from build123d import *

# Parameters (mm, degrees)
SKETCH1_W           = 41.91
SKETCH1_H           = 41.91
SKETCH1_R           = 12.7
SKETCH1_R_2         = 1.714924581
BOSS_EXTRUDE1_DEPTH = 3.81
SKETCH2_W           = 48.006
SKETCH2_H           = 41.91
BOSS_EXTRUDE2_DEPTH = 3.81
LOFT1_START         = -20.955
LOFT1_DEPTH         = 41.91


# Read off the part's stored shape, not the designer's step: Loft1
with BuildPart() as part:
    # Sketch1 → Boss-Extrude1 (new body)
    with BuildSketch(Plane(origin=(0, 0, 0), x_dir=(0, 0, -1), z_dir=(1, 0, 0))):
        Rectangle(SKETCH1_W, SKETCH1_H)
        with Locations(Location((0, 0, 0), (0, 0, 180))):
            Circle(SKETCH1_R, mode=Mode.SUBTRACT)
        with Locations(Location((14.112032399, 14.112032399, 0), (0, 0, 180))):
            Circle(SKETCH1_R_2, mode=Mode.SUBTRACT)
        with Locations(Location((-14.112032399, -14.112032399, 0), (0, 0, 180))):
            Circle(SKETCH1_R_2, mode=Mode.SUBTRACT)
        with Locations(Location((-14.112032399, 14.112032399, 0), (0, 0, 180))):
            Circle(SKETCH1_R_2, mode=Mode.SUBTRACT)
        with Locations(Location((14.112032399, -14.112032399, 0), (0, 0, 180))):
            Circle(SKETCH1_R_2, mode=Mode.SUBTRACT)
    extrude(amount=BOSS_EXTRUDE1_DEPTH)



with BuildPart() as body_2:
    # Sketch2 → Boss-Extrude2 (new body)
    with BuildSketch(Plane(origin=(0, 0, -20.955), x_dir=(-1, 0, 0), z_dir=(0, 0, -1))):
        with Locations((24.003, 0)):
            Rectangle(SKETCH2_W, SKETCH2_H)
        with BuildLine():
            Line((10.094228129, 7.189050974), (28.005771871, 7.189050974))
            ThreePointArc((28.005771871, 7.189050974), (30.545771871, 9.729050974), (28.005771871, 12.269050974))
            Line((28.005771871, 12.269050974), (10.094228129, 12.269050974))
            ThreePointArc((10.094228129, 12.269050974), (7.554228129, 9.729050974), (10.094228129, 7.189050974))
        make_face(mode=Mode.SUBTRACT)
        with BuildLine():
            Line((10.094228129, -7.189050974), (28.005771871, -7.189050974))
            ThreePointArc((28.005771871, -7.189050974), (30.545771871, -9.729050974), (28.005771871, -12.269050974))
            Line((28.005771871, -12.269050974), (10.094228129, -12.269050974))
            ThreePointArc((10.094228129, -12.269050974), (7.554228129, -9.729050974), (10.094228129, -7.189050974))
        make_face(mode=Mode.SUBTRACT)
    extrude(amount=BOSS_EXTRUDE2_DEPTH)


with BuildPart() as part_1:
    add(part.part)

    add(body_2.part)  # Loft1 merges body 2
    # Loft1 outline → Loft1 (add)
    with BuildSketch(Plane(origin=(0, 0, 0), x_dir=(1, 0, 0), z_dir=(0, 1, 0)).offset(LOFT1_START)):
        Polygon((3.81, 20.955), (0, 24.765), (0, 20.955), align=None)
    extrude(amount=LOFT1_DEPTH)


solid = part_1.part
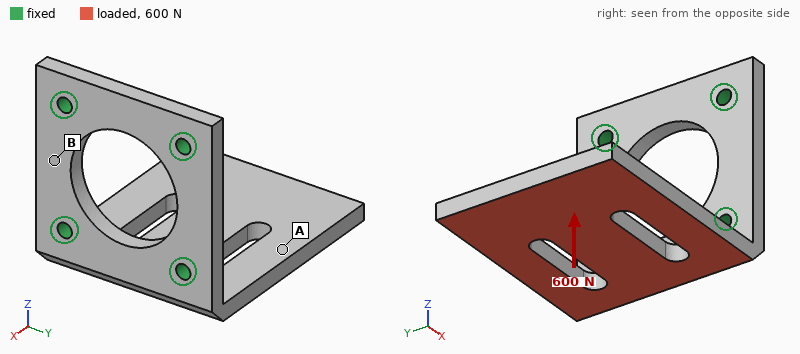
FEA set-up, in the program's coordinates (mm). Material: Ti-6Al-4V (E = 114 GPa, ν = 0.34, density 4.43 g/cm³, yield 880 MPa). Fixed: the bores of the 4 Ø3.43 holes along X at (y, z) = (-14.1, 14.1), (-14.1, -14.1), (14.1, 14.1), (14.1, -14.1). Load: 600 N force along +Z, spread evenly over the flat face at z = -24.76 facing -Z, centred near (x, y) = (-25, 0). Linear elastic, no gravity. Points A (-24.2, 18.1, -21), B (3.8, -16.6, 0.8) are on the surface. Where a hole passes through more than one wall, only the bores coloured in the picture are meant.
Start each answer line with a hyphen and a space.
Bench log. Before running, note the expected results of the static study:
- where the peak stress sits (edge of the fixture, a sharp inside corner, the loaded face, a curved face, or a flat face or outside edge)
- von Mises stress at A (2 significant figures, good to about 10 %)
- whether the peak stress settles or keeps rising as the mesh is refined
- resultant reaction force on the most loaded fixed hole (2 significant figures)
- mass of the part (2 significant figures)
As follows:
- edge of the fixture
- 49 MPa
- keeps rising
- 340 N
- 52 g
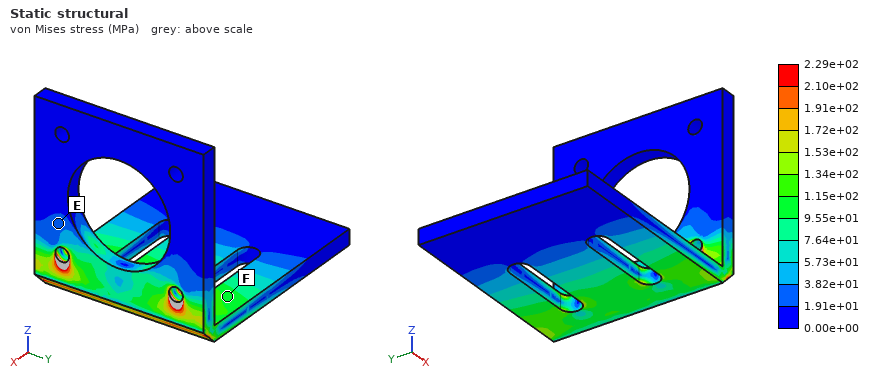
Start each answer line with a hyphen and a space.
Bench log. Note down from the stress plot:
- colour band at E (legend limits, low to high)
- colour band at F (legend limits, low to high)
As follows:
- 1.91e+01 to 3.82e+01 MPa
- 9.55e+01 to 1.15e+02 MPa
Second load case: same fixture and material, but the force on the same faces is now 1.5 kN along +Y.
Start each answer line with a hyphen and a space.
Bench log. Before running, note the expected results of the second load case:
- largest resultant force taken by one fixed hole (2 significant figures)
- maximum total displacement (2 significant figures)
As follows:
- 1.6 kN
- 0.12 mm
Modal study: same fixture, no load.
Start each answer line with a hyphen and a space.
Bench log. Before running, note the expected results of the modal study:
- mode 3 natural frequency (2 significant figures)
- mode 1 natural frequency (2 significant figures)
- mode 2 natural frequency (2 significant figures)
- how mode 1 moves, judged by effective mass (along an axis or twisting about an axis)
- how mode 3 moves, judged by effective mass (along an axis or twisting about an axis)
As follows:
- 3900 Hz
- 910 Hz
- 2700 Hz
- along Z
- along Y
